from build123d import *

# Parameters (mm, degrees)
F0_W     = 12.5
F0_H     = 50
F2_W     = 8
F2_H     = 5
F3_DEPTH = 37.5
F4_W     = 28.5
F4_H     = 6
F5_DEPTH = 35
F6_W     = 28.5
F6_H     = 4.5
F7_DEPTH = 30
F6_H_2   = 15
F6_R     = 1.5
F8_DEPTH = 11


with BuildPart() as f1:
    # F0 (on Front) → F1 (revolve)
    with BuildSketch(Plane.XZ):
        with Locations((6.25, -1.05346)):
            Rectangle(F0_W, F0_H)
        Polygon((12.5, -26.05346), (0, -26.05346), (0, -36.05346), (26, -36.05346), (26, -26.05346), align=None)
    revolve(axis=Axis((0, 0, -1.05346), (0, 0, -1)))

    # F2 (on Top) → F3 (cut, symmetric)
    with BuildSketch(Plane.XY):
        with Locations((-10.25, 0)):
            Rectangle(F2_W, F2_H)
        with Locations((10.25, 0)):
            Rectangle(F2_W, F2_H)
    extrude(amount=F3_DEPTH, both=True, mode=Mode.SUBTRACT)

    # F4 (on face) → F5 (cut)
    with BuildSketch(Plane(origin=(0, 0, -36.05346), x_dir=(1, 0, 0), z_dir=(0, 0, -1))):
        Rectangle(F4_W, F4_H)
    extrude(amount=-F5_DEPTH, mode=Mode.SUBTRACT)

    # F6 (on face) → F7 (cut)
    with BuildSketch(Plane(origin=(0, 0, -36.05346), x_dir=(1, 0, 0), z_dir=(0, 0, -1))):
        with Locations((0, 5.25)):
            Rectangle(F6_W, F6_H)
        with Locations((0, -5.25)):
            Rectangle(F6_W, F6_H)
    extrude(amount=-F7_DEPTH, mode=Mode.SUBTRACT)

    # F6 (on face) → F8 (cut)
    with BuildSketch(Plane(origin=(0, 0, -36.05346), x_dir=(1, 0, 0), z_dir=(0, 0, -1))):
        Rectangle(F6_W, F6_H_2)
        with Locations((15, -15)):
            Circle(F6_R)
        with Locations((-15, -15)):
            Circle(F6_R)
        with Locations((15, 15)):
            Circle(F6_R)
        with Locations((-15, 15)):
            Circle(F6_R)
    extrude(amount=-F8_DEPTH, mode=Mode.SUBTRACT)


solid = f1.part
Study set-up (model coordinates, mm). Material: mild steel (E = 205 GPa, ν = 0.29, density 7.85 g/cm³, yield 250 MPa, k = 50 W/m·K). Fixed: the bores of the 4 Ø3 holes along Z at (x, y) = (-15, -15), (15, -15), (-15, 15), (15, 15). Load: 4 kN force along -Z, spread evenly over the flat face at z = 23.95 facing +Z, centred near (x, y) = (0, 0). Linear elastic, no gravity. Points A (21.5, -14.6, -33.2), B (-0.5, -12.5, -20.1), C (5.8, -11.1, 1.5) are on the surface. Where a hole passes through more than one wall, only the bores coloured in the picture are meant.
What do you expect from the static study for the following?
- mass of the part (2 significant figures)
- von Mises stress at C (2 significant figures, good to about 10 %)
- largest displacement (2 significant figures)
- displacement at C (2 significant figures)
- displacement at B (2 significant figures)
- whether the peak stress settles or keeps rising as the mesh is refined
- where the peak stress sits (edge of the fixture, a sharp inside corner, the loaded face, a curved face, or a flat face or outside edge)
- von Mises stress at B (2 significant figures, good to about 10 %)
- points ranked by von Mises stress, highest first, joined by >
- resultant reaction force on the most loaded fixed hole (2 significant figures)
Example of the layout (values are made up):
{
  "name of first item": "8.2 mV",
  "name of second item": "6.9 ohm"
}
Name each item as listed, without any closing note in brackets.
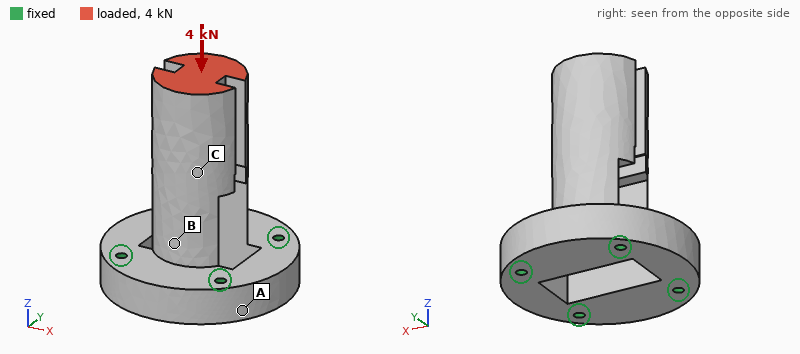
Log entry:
{
  "mass of the part": "250 g",
  "von Mises stress at C": "22 MPa",
  "largest displacement": "7.8 µm",
  "displacement at C": "6.4 µm",
  "displacement at B": "4.2 µm",
  "whether the peak stress settles or keeps rising as the mesh is refined": "keeps rising",
  "where the peak stress sits": "edge of the fixture",
  "von Mises stress at B": "38 MPa",
  "points ranked by von Mises stress, highest first, joined by >": "B > C > A",
  "resultant reaction force on the most loaded fixed hole": "1.0 kN"
}
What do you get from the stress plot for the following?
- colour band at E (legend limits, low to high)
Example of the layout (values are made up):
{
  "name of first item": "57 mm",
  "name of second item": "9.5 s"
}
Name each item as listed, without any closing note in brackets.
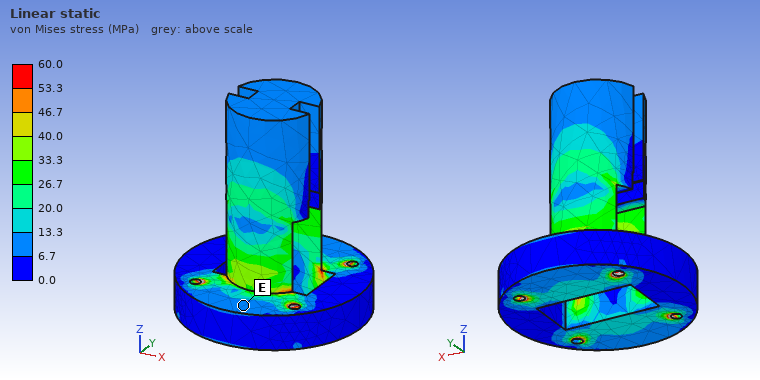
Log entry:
{
  "colour band at E": "6.7 to 13.3 MPa"
}
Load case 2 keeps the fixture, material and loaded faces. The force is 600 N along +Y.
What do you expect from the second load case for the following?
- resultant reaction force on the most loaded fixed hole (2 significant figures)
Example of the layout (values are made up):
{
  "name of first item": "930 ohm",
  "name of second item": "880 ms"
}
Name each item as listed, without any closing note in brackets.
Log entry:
{
  "resultant reaction force on the most loaded fixed hole": "610 N"
}
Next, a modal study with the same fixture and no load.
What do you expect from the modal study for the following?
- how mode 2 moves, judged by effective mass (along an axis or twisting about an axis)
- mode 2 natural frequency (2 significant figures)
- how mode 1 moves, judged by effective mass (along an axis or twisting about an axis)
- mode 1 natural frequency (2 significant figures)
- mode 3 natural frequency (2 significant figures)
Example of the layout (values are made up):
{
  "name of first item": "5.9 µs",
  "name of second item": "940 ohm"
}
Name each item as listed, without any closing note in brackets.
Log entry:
{
  "how mode 2 moves, judged by effective mass": "along Y",
  "mode 2 natural frequency": "2600 Hz",
  "how mode 1 moves, judged by effective mass": "along X",
  "mode 1 natural frequency": "2400 Hz",
  "mode 3 natural frequency": "6900 Hz"
}
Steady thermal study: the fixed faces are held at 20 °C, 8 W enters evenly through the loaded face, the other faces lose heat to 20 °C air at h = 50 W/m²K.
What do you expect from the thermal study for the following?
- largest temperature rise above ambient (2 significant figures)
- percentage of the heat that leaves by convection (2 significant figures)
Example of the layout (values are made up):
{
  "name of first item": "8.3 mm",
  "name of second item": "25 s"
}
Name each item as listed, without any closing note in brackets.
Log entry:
{
  "largest temperature rise above ambient": "25 K",
  "percentage of the heat that leaves by convection": "54 %"
}
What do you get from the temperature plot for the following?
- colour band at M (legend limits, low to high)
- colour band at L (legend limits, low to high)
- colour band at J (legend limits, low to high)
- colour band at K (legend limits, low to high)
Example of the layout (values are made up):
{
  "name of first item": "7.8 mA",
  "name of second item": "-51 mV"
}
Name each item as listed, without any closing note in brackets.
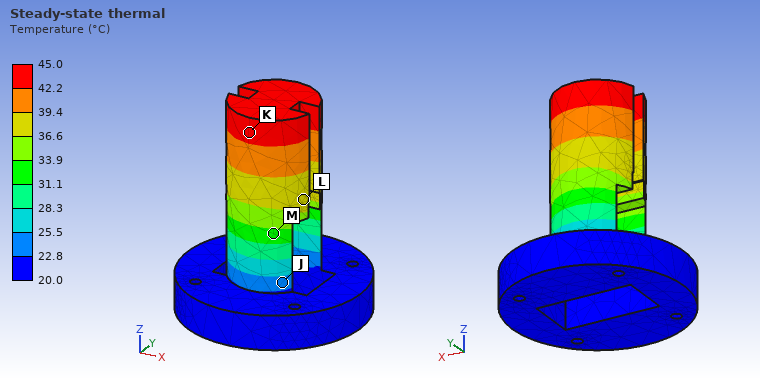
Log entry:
{
  "colour band at M": "31.1 to 33.9 °C",
  "colour band at L": "36.6 to 39.4 °C",
  "colour band at J": "22.8 to 25.5 °C",
  "colour band at K": "42.2 to 45.0 °C"
}
